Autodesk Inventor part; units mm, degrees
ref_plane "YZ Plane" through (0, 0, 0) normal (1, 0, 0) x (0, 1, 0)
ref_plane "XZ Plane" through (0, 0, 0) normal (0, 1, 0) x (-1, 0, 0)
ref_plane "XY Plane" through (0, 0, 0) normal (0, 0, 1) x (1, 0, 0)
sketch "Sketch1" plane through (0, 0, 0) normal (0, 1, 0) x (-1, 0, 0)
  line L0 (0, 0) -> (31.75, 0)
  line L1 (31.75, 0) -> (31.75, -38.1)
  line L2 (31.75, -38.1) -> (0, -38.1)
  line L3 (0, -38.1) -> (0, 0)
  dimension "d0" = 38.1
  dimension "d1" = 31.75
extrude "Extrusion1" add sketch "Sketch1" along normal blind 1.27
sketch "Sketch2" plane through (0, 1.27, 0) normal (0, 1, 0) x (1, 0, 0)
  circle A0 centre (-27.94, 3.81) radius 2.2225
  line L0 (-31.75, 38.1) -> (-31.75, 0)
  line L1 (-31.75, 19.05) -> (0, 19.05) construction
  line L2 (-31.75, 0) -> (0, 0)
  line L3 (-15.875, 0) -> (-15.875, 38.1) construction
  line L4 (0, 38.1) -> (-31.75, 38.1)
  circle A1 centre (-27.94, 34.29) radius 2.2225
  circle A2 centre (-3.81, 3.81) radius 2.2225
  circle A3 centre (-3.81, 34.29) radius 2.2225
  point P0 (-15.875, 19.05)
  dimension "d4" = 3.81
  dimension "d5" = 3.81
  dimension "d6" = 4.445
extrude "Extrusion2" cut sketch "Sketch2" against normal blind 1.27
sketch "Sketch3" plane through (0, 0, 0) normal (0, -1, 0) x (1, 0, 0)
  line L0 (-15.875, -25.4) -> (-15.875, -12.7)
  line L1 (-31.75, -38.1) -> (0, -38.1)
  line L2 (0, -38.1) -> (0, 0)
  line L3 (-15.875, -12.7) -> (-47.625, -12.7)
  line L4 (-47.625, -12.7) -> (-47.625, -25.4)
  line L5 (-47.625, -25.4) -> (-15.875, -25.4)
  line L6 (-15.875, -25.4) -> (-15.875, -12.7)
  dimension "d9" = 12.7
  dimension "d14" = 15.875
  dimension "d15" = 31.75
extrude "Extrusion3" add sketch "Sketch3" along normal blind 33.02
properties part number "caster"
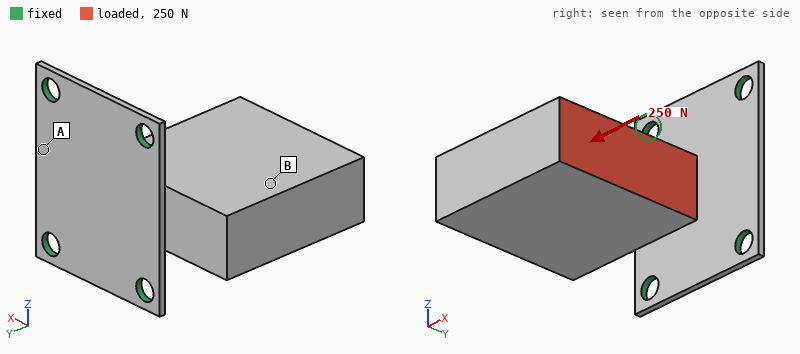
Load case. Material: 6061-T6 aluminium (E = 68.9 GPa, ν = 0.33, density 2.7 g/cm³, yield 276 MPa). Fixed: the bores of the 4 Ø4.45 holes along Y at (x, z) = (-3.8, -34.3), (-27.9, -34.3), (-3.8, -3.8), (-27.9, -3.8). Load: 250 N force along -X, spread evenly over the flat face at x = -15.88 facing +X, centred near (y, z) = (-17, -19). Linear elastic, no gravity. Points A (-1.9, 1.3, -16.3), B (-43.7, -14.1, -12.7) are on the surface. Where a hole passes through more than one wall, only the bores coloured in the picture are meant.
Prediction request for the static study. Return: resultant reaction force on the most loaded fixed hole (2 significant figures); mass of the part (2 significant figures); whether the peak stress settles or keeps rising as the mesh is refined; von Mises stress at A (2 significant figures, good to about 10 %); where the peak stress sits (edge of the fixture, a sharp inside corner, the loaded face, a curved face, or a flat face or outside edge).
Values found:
140 N
40 g
keeps rising
42 MPa
edge of the fixture
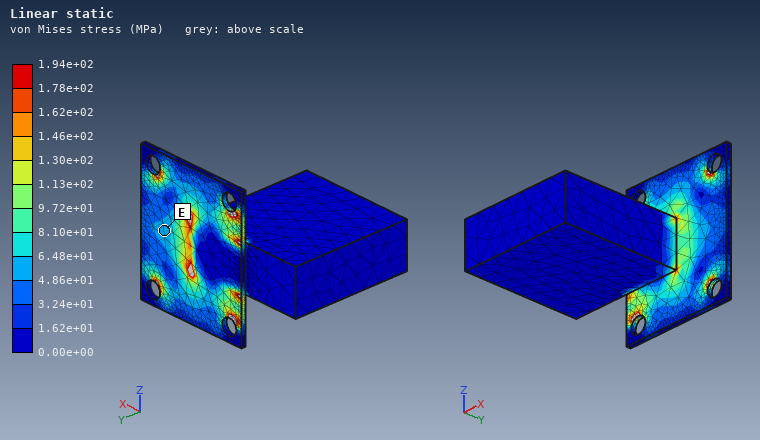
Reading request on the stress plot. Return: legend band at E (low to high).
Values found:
4.86e+01 to 6.48e+01 MPa
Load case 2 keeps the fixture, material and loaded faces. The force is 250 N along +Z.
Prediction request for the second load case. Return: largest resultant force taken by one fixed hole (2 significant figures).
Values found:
190 N
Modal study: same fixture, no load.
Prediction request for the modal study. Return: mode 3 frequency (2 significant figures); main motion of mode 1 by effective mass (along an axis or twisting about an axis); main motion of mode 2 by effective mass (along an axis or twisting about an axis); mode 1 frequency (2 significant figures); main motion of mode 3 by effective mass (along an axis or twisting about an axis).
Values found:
2400 Hz
along X
along Z
700 Hz
along Y
